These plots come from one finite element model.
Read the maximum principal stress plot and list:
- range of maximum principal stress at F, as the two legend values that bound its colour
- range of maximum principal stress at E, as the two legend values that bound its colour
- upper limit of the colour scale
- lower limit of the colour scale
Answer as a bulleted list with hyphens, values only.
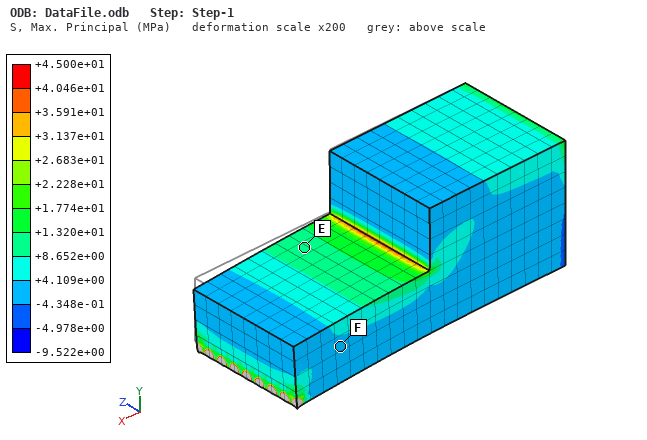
- -4.348e-01 to +4.109e+00 MPa
- +8.652e+00 to +1.320e+01 MPa
- +4.500e+01 MPa
- -9.522e+00 MPa
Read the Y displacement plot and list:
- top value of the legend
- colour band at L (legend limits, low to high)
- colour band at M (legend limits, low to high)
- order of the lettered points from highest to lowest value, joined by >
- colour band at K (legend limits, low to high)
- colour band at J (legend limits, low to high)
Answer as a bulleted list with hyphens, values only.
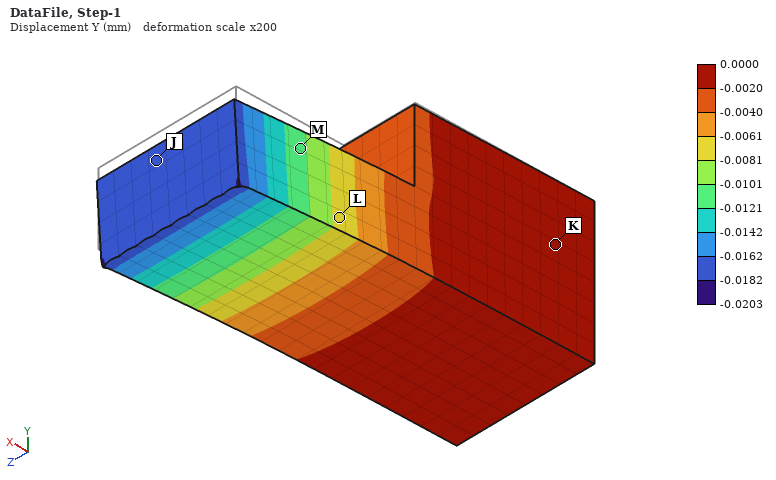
- 0.0000 mm
- -0.0081 to -0.0061 mm
- -0.0121 to -0.0101 mm
- K > L > M > J
- -0.0020 to 0.0000 mm
- -0.0182 to -0.0162 mm
